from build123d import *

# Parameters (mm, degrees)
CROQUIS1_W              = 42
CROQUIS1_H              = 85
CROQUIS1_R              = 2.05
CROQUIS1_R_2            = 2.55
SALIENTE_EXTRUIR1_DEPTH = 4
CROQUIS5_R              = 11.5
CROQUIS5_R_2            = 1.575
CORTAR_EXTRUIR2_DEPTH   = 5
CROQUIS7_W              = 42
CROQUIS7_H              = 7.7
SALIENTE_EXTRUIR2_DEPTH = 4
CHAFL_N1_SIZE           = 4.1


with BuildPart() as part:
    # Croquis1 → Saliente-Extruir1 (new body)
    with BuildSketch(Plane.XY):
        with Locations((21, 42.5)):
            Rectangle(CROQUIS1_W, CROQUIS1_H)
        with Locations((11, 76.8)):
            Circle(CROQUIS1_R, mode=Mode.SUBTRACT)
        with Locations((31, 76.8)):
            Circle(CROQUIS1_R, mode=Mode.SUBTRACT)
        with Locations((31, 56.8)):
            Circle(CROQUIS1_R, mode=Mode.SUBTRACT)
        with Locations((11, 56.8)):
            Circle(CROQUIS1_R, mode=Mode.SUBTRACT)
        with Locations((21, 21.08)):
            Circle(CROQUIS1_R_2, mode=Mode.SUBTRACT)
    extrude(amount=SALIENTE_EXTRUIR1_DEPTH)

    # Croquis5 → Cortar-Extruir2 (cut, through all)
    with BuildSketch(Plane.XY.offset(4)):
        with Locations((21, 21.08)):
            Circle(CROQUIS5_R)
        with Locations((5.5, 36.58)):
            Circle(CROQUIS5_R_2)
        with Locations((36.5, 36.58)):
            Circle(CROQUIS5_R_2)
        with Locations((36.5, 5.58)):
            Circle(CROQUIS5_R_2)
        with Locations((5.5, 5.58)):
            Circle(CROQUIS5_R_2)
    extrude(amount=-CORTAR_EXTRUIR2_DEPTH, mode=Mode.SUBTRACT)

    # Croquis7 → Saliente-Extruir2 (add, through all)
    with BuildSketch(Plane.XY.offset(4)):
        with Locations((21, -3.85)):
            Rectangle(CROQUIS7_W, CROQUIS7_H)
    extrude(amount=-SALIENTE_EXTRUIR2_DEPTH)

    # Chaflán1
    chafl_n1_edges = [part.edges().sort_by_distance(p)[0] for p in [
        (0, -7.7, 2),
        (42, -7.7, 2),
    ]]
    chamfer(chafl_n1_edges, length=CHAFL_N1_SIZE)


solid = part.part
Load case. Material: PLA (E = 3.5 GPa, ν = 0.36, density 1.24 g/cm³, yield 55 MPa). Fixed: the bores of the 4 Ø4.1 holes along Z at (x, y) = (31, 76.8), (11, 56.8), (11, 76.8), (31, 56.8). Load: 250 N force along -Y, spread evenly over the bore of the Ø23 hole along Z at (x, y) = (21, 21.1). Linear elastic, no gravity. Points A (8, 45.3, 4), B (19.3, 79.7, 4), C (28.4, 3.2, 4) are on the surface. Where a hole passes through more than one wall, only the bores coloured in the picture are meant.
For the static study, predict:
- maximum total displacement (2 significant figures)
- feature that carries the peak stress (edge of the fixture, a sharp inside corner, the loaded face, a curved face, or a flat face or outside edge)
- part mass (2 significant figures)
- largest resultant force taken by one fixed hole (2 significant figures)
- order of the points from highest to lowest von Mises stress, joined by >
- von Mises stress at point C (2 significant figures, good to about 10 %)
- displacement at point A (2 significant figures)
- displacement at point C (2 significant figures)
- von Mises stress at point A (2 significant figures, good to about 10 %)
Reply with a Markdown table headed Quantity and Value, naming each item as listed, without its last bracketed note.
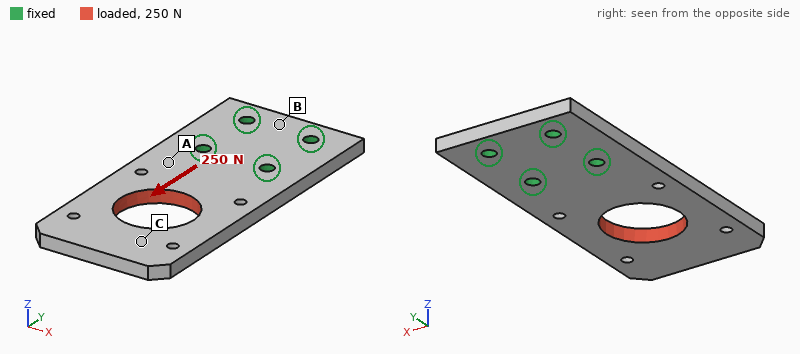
| Quantity | Value |
|---|---|
| maximum total displacement | 35 µm |
| feature that carries the peak stress | a curved face |
| part mass | 17 g |
| largest resultant force taken by one fixed hole | 100 N |
| order of the points from highest to lowest von Mises stress, joined by > | A > C > B |
| von Mises stress at point C | 0.94 MPa |
| displacement at point A | 6.8 µm |
| displacement at point C | 31 µm |
| von Mises stress at point A | 1.7 MPa |
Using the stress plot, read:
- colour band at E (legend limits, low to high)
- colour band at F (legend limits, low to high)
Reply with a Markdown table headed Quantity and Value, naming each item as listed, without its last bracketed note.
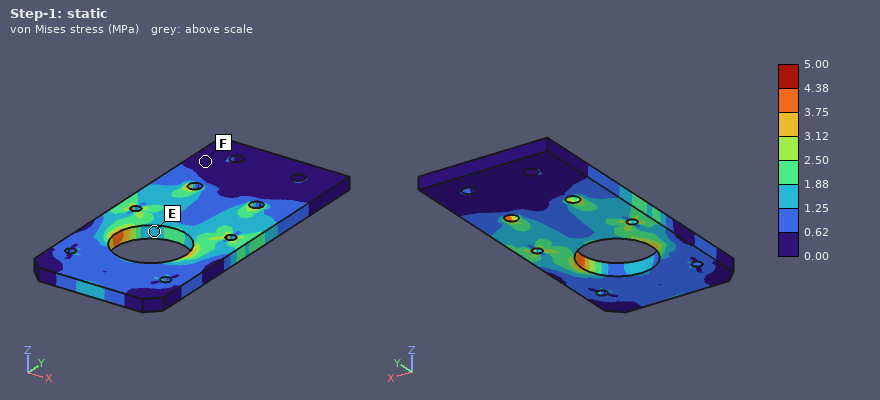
| Quantity | Value |
|---|---|
| colour band at E | 1.25 to 1.88 MPa |
| colour band at F | 0.00 to 0.62 MPa |
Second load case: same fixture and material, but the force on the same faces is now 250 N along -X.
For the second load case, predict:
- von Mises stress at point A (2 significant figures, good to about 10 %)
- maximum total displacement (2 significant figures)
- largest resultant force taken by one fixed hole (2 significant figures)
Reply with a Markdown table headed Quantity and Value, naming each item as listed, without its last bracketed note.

| Quantity | Value |
|---|---|
| von Mises stress at point A | 3.2 MPa |
| maximum total displacement | 0.28 mm |
| largest resultant force taken by one fixed hole | 310 N |
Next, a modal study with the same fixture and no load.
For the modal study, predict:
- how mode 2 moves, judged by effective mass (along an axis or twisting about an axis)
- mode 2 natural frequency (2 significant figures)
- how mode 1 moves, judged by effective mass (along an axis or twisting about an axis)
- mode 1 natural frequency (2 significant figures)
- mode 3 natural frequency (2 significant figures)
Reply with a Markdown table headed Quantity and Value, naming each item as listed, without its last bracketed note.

| Quantity | Value |
|---|---|
| how mode 2 moves, judged by effective mass | twisting about Y |
| mode 2 natural frequency | 780 Hz |
| how mode 1 moves, judged by effective mass | along Z |
| mode 1 natural frequency | 260 Hz |
| mode 3 natural frequency | 1500 Hz |
